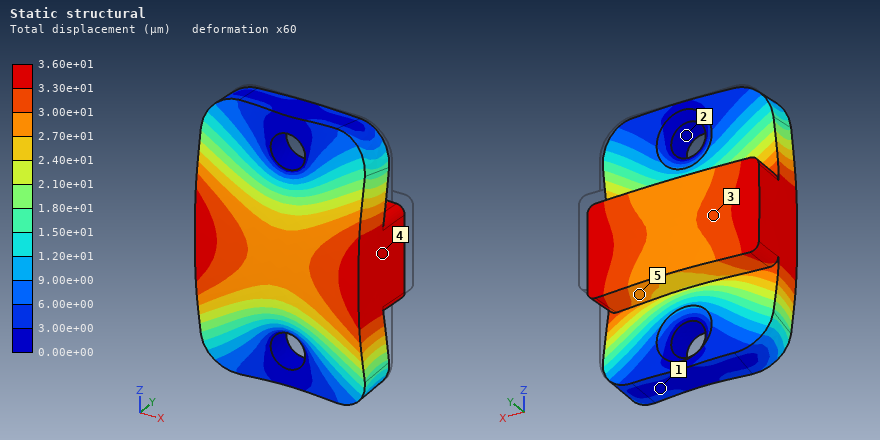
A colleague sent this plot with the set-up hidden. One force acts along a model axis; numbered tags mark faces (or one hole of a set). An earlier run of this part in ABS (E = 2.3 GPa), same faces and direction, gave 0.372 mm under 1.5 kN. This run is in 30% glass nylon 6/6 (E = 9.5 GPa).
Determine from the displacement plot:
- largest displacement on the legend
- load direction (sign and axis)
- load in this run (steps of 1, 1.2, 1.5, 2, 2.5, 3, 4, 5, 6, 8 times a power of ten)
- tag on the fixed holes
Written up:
3.60e+01 µm
-Y
600 N
2
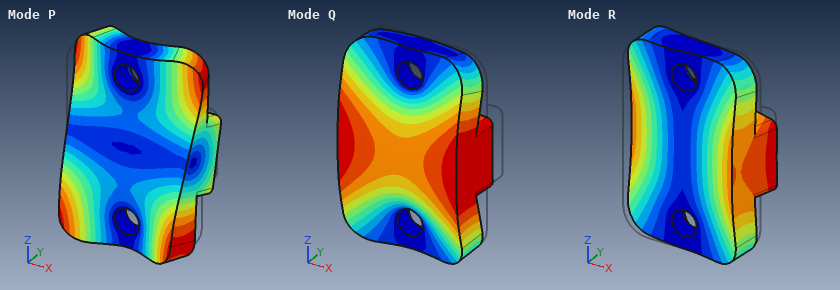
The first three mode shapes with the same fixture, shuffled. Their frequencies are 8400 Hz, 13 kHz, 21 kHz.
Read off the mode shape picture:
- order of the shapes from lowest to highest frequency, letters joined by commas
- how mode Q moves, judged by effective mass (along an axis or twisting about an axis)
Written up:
R, Q, P
along Y
